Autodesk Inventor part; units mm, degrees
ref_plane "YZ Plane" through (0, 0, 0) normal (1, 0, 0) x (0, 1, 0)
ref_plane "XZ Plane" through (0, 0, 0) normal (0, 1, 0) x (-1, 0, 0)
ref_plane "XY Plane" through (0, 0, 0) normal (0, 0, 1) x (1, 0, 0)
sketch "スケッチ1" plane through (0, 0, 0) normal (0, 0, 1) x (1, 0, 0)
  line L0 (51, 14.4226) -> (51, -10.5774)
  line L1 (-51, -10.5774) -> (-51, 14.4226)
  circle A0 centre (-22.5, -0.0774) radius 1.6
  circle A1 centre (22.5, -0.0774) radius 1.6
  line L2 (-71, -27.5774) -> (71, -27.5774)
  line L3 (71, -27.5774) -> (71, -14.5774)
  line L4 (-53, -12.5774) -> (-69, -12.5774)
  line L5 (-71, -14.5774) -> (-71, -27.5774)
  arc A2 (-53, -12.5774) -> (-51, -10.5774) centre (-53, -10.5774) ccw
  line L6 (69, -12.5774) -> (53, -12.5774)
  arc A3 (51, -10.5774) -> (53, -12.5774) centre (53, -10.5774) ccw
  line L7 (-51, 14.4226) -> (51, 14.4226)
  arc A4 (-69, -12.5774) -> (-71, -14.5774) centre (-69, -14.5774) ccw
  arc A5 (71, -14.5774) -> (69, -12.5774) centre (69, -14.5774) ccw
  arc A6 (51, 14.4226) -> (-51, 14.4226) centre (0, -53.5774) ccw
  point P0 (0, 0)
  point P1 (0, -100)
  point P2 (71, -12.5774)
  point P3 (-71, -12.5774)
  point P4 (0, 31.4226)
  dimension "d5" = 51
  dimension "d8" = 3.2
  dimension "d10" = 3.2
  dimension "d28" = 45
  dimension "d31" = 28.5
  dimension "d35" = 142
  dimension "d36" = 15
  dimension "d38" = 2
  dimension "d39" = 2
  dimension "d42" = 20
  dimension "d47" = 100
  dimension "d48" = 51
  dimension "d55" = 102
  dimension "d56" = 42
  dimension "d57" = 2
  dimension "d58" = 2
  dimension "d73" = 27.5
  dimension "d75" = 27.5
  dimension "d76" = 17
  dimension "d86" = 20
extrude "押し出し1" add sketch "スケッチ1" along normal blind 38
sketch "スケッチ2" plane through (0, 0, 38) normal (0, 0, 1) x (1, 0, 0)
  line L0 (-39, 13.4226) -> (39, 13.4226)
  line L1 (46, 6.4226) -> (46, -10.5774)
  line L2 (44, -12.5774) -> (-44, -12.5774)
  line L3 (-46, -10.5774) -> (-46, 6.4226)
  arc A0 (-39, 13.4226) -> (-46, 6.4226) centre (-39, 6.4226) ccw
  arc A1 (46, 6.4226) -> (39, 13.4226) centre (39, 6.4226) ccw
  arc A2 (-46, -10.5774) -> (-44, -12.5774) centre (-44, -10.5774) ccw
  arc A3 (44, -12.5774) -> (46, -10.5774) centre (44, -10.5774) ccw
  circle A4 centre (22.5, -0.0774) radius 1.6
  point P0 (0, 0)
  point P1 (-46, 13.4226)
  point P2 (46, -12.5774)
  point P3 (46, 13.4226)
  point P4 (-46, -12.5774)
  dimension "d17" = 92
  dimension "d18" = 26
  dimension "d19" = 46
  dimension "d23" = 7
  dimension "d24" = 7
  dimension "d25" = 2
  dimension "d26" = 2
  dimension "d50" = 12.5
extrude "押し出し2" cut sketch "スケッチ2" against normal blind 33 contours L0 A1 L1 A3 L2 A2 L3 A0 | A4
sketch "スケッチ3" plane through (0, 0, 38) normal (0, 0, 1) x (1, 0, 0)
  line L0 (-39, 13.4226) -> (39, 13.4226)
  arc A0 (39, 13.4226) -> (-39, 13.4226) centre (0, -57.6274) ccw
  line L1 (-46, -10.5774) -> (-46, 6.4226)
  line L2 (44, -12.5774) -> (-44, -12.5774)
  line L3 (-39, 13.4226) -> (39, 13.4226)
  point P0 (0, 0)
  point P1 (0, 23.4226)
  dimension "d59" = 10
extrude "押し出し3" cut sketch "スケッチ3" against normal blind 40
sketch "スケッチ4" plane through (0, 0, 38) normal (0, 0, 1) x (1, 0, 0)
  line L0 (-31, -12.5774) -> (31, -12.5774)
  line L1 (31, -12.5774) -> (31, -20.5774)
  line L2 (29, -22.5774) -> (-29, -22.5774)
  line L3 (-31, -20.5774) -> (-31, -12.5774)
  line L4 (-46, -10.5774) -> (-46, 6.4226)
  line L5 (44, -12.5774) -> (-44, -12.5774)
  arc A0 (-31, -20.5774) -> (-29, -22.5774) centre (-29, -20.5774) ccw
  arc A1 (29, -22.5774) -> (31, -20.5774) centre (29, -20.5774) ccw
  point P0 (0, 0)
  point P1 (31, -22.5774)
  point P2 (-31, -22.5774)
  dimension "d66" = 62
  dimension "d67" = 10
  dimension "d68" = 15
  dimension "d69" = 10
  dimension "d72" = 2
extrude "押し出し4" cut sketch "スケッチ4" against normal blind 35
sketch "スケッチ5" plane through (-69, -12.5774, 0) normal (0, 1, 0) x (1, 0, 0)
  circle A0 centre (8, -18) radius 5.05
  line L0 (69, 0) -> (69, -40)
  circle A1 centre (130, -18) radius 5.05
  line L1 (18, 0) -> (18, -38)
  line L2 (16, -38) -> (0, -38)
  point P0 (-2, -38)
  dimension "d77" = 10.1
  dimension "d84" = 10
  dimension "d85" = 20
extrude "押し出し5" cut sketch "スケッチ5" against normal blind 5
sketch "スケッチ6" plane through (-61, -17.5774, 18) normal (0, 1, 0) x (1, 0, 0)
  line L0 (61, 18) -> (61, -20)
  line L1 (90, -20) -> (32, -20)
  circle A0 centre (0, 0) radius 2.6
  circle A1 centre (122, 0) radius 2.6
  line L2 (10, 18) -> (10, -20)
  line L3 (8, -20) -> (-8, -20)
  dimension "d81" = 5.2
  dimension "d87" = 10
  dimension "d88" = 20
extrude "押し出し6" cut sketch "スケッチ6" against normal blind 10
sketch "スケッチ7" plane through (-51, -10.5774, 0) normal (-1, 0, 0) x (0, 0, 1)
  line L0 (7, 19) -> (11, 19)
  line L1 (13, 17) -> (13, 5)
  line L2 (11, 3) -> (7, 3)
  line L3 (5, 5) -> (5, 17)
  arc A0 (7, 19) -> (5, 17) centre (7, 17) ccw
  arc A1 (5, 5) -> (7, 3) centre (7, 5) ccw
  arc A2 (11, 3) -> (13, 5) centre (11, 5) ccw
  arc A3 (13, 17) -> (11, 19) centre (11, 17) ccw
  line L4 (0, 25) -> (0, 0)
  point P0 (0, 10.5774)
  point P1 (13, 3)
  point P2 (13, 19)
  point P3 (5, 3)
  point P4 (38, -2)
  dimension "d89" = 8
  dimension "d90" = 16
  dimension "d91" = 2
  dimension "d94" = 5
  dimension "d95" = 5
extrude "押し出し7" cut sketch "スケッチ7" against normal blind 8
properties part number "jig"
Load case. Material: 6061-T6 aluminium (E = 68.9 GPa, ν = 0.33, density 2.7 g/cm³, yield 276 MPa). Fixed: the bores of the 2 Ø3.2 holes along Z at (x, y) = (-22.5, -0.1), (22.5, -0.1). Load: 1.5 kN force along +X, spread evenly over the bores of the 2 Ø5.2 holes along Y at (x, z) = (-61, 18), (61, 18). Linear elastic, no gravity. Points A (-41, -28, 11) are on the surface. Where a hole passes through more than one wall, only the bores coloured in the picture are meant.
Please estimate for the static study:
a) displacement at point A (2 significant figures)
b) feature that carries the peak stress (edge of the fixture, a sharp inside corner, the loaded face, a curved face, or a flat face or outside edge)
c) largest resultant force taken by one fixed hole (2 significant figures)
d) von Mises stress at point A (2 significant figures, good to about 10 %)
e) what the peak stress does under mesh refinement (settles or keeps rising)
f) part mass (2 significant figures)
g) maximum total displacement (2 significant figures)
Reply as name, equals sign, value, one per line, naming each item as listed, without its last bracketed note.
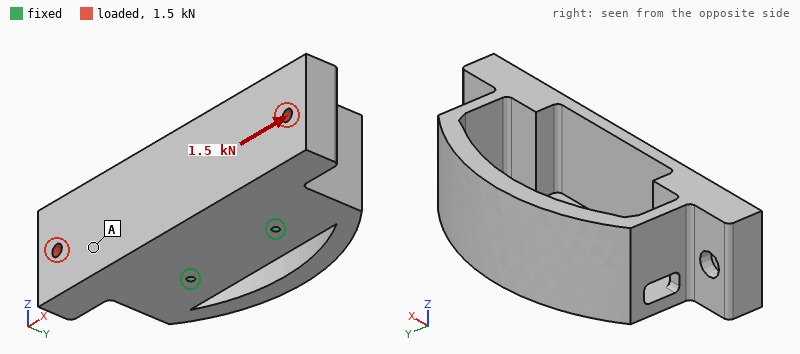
displacement at point A = 36 µm
feature that carries the peak stress = edge of the fixture
largest resultant force taken by one fixed hole = 1.1 kN
von Mises stress at point A = 4.2 MPa
what the peak stress does under mesh refinement = keeps rising
part mass = 290 g
maximum total displacement = 68 µm
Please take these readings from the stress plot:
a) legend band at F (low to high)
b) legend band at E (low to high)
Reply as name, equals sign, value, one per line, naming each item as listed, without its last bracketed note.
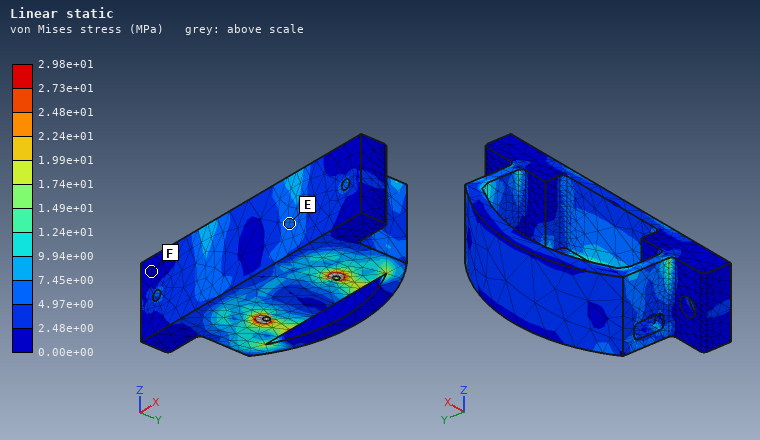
legend band at F = 0.00e+00 to 2.48e+00 MPa
legend band at E = 4.97e+00 to 7.45e+00 MPa
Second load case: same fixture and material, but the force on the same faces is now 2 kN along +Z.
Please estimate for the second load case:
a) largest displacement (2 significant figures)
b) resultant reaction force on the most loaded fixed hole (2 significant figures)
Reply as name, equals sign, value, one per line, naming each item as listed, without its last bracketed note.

largest displacement = 0.43 mm
resultant reaction force on the most loaded fixed hole = 1.0 kN
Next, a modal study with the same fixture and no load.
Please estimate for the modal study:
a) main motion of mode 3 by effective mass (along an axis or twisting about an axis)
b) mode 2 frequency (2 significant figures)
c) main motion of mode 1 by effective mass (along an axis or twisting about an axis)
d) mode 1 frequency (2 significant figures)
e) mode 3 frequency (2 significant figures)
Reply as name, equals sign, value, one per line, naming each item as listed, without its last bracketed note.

main motion of mode 3 by effective mass = along Z
mode 2 frequency = 1300 Hz
main motion of mode 1 by effective mass = along Y
mode 1 frequency = 710 Hz
mode 3 frequency = 2100 Hz
